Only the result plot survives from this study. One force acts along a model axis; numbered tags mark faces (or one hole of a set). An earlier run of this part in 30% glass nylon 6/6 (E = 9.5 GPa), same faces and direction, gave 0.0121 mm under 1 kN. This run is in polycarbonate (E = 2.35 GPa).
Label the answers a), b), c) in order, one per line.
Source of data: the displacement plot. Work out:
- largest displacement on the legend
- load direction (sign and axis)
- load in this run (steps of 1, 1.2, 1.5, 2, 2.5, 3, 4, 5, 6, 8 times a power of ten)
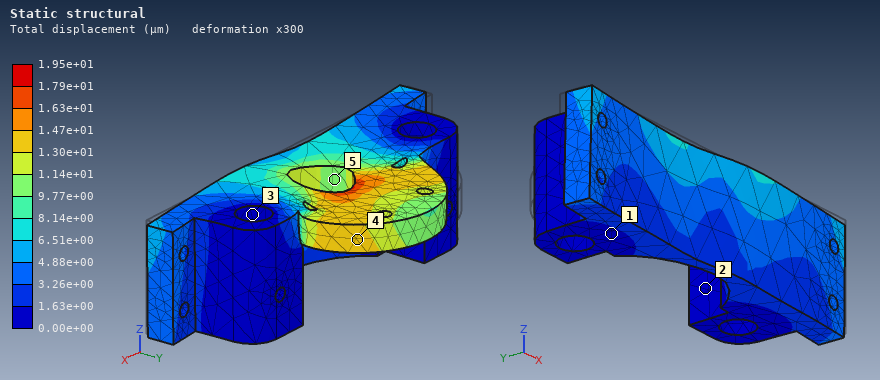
a) 1.95e+01 µm
b) +X
c) 400 N
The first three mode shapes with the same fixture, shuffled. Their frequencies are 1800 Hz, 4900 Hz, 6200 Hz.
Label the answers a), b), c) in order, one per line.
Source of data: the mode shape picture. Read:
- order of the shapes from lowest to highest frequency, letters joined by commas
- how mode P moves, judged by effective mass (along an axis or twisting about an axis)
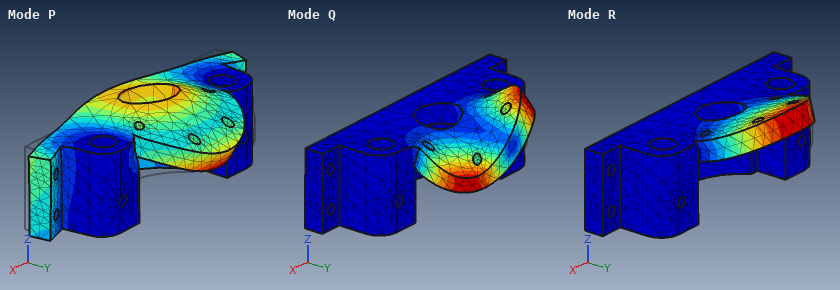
a) R, Q, P
b) along Y
